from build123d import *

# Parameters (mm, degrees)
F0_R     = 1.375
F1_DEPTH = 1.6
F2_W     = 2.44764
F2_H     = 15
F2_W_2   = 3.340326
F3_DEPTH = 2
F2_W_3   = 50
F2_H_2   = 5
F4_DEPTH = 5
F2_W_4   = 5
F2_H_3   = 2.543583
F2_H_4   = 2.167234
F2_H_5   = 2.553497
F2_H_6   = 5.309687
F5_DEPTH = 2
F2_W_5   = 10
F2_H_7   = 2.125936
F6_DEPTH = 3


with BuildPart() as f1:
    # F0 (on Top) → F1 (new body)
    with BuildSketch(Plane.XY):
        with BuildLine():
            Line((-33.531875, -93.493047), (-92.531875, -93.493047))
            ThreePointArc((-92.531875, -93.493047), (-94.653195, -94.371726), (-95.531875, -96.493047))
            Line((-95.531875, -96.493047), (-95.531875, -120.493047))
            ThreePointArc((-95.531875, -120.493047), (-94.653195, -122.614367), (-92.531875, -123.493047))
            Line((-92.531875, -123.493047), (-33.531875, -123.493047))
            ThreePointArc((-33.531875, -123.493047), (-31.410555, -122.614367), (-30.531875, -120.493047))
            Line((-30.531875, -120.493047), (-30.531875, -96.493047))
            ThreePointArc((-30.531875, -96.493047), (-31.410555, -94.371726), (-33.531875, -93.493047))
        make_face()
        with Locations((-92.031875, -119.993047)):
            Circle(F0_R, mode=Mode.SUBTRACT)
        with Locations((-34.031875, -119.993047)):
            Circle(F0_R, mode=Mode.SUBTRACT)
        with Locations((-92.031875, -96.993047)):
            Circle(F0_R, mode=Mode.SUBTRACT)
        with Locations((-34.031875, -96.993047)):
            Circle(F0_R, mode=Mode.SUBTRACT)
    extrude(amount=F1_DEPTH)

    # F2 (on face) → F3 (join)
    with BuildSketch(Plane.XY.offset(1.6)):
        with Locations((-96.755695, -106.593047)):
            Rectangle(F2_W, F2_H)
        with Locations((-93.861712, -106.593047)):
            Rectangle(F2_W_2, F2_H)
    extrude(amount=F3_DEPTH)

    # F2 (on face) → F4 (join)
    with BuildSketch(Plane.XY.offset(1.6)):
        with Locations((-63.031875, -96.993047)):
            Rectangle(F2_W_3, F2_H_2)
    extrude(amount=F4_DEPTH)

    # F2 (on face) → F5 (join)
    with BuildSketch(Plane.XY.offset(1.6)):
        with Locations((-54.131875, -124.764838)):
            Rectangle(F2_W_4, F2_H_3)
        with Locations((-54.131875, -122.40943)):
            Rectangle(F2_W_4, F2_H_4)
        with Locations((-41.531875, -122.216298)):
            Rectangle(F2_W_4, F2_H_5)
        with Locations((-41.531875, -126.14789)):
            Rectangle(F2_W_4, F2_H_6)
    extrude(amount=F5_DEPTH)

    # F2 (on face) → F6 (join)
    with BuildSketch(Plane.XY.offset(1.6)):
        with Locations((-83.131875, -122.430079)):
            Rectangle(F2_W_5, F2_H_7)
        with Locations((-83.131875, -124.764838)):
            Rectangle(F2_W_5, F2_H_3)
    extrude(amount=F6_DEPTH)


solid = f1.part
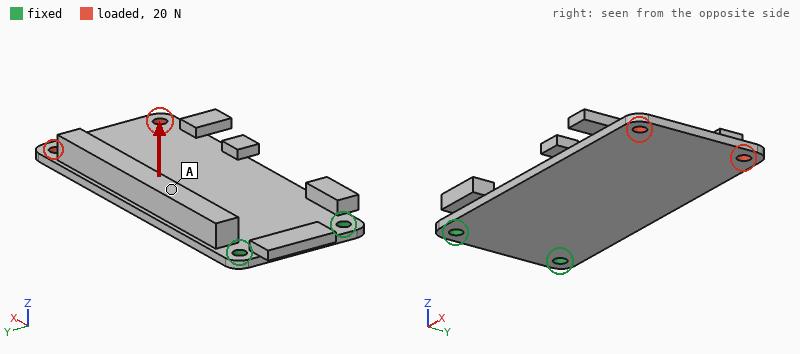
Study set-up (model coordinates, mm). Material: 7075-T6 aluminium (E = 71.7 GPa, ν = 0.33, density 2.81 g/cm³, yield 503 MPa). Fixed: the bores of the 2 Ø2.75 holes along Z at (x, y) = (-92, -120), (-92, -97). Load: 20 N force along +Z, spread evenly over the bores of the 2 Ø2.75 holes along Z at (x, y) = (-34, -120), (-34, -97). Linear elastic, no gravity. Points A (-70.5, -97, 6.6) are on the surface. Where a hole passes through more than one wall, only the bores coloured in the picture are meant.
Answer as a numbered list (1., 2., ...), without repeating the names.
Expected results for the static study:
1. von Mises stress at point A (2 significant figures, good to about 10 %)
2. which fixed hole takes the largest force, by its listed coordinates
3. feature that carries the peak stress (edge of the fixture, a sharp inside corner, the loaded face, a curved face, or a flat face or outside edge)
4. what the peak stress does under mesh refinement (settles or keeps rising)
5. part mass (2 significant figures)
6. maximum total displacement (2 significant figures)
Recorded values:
1. 15 MPa
2. (-92, -120)
3. edge of the fixture
4. keeps rising
5. 13 g
6. 0.75 mm
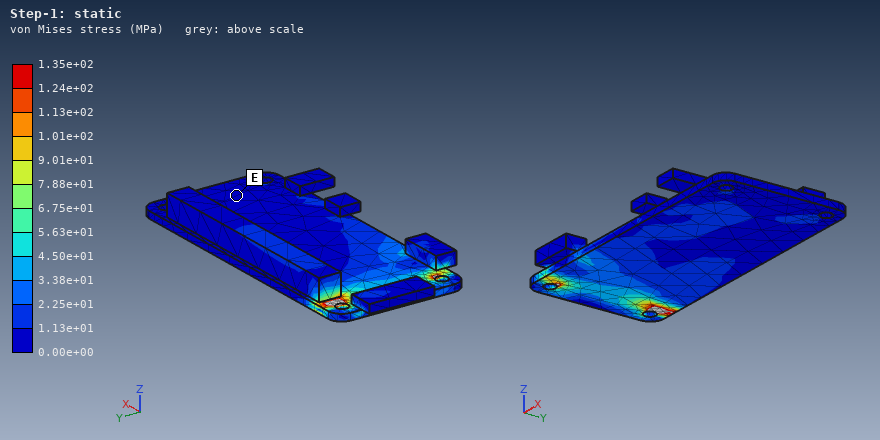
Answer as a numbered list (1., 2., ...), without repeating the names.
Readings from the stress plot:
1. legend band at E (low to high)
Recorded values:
1. 0.00e+00 to 1.13e+01 MPa
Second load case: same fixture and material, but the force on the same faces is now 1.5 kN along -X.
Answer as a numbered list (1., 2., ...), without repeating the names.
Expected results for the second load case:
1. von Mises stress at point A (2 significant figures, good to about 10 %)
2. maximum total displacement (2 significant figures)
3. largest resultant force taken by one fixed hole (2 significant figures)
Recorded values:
1. 11 MPa
2. 0.16 mm
3. 760 N
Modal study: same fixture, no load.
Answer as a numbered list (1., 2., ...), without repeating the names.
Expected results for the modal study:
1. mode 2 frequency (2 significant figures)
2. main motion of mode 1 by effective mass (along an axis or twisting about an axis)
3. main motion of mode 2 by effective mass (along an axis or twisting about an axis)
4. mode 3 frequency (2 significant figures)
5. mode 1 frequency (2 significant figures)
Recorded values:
1. 1700 Hz
2. along Z
3. twisting about X
4. 3600 Hz
5. 440 Hz
